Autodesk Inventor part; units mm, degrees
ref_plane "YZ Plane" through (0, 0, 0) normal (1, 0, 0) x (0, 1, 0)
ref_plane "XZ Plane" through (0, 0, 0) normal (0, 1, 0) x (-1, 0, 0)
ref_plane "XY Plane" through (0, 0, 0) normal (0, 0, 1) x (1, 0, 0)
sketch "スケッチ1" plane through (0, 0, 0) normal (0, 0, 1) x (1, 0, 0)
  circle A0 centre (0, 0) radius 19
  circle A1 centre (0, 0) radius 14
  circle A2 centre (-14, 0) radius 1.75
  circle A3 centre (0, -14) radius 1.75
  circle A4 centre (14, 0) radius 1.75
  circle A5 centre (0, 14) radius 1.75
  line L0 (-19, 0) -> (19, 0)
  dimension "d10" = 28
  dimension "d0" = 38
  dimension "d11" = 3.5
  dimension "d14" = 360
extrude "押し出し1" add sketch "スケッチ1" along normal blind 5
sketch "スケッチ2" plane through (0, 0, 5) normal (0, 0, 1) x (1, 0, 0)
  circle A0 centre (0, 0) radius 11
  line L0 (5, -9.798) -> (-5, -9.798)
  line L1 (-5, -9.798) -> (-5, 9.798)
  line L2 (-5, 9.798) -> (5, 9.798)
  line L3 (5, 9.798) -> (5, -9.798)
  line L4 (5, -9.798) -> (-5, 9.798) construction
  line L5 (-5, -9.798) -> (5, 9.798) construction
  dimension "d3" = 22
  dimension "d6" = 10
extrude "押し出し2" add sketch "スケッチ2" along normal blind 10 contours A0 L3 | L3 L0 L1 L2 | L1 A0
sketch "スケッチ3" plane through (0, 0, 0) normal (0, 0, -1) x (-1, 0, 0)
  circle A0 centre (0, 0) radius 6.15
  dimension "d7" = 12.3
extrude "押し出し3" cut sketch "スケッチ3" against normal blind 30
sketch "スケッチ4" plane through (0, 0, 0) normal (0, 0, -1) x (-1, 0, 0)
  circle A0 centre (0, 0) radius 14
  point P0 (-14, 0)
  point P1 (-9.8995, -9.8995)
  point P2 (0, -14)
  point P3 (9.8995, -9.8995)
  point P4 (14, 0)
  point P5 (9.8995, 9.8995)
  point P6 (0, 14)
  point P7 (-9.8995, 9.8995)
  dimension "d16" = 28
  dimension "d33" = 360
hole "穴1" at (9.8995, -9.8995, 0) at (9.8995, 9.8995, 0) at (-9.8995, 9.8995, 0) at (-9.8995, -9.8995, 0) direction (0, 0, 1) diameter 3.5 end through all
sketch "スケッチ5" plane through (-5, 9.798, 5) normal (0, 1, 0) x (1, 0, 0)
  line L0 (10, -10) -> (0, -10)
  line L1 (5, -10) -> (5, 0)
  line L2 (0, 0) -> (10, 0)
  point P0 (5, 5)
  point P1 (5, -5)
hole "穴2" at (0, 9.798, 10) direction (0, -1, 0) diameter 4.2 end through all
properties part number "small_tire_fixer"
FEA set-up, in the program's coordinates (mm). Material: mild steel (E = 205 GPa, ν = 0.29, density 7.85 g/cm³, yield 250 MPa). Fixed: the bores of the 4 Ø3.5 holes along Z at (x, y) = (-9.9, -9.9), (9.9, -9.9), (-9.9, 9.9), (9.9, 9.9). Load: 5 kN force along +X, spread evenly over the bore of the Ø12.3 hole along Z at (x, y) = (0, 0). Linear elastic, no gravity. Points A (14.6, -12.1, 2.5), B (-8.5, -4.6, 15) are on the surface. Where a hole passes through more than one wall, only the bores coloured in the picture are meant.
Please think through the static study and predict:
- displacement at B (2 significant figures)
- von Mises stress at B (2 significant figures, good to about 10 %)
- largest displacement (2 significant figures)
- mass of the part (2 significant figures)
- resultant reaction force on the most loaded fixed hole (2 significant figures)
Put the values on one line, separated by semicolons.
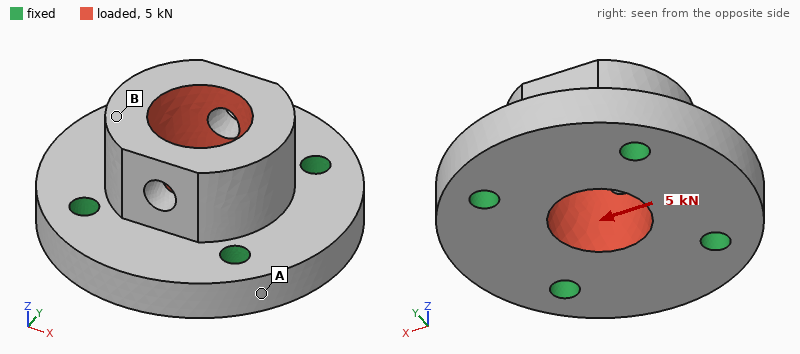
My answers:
4.7 µm; 16 MPa; 5.1 µm; 57 g; 1.4 kN
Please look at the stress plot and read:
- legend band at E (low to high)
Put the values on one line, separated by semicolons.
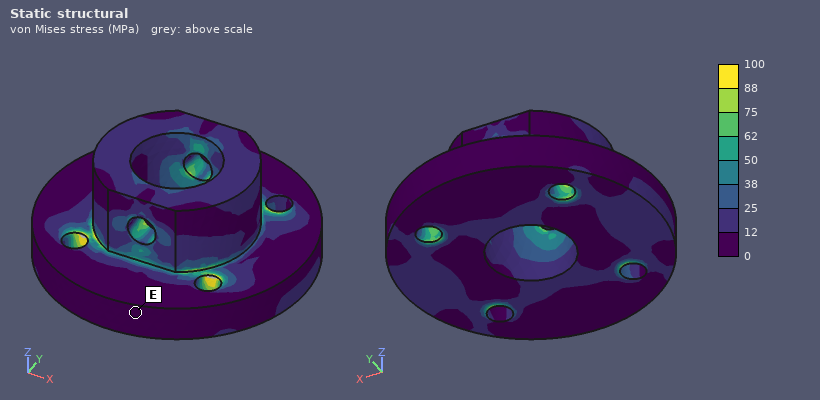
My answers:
0 to 12 MPa
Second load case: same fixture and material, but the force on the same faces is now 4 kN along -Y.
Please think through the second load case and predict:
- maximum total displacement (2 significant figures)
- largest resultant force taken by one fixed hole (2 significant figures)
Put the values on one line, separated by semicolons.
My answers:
3.6 µm; 1.1 kN
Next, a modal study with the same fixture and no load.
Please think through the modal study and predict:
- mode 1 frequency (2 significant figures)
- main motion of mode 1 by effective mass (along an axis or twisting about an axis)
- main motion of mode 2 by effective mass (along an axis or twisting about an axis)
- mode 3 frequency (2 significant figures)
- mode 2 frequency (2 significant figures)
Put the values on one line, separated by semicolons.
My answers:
33 kHz; along X; along Y; 39 kHz; 36 kHz
